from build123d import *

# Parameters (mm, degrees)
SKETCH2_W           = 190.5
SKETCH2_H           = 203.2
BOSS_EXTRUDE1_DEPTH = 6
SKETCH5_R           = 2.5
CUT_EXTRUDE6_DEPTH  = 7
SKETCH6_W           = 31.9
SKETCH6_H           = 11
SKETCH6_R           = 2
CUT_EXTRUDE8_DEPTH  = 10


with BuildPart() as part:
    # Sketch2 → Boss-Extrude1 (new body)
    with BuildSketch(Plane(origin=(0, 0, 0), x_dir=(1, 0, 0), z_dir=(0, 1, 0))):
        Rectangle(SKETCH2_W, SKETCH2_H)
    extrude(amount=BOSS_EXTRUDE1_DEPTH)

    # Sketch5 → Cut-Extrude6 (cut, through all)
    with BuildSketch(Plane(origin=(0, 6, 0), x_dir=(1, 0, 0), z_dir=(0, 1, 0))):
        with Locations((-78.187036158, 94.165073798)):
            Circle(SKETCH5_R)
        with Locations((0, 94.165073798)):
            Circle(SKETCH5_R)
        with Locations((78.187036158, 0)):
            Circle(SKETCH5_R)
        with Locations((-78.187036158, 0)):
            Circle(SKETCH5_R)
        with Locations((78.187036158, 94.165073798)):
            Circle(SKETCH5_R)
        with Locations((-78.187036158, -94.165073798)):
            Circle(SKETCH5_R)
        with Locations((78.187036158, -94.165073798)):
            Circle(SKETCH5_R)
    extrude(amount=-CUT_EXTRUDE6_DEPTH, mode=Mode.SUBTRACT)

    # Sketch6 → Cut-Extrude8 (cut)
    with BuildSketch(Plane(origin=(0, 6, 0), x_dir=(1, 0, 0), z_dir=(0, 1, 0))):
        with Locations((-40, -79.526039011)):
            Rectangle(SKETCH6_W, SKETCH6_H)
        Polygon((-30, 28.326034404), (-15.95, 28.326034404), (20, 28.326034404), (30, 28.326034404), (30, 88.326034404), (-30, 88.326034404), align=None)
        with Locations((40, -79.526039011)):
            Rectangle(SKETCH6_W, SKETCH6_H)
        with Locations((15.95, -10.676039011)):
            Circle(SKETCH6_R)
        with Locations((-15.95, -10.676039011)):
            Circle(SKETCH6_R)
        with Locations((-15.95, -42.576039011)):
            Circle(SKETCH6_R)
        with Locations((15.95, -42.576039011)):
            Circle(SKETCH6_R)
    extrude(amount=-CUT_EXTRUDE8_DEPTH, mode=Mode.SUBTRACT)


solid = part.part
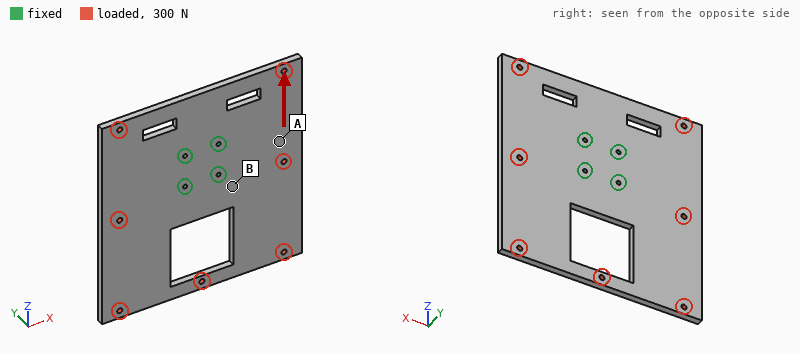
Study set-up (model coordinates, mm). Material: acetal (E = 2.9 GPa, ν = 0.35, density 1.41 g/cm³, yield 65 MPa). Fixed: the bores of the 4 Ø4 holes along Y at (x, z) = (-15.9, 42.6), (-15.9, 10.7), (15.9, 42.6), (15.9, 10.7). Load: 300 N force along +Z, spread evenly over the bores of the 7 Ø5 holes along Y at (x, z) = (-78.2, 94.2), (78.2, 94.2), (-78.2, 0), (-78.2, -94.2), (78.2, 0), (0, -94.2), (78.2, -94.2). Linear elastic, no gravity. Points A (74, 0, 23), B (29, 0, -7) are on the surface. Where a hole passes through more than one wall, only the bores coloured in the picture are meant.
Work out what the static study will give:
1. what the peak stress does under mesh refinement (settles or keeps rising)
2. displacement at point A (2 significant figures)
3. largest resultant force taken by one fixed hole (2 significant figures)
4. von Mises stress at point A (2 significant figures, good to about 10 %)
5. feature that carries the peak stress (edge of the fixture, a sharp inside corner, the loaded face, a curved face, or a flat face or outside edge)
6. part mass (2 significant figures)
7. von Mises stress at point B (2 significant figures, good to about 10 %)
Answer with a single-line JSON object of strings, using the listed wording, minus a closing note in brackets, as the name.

{"what the peak stress does under mesh refinement": "keeps rising", "displacement at point A": "16 µm", "largest resultant force taken by one fixed hole": "83 N", "von Mises stress at point A": "0.18 MPa", "feature that carries the peak stress": "edge of the fixture", "part mass": "290 g", "von Mises stress at point B": "0.55 MPa"}
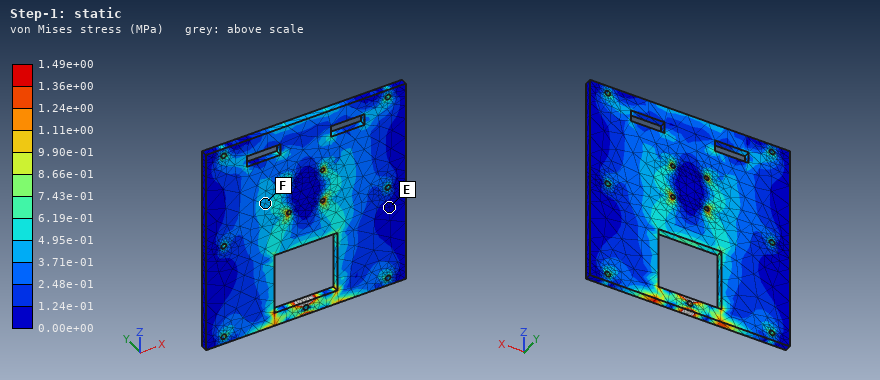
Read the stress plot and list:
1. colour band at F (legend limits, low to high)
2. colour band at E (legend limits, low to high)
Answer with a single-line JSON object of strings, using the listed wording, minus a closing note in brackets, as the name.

{"colour band at F": "3.71e-01 to 4.95e-01 MPa", "colour band at E": "0.00e+00 to 1.24e-01 MPa"}
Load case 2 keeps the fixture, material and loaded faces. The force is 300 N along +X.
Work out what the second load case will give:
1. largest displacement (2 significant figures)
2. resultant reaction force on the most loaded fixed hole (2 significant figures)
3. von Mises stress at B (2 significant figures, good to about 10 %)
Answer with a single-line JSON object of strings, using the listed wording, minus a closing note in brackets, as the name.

{"largest displacement": "0.13 mm", "resultant reaction force on the most loaded fixed hole": "200 N", "von Mises stress at B": "0.54 MPa"}
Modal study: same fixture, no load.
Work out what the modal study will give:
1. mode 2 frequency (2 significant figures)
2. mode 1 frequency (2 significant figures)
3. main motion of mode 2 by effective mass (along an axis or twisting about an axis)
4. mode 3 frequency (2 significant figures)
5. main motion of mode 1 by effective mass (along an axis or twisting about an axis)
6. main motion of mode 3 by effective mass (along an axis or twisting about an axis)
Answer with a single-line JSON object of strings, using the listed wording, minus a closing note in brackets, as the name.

{"mode 2 frequency": "110 Hz", "mode 1 frequency": "90 Hz", "main motion of mode 2 by effective mass": "twisting about Z", "mode 3 frequency": "190 Hz", "main motion of mode 1 by effective mass": "along Y", "main motion of mode 3 by effective mass": "along Y"}
